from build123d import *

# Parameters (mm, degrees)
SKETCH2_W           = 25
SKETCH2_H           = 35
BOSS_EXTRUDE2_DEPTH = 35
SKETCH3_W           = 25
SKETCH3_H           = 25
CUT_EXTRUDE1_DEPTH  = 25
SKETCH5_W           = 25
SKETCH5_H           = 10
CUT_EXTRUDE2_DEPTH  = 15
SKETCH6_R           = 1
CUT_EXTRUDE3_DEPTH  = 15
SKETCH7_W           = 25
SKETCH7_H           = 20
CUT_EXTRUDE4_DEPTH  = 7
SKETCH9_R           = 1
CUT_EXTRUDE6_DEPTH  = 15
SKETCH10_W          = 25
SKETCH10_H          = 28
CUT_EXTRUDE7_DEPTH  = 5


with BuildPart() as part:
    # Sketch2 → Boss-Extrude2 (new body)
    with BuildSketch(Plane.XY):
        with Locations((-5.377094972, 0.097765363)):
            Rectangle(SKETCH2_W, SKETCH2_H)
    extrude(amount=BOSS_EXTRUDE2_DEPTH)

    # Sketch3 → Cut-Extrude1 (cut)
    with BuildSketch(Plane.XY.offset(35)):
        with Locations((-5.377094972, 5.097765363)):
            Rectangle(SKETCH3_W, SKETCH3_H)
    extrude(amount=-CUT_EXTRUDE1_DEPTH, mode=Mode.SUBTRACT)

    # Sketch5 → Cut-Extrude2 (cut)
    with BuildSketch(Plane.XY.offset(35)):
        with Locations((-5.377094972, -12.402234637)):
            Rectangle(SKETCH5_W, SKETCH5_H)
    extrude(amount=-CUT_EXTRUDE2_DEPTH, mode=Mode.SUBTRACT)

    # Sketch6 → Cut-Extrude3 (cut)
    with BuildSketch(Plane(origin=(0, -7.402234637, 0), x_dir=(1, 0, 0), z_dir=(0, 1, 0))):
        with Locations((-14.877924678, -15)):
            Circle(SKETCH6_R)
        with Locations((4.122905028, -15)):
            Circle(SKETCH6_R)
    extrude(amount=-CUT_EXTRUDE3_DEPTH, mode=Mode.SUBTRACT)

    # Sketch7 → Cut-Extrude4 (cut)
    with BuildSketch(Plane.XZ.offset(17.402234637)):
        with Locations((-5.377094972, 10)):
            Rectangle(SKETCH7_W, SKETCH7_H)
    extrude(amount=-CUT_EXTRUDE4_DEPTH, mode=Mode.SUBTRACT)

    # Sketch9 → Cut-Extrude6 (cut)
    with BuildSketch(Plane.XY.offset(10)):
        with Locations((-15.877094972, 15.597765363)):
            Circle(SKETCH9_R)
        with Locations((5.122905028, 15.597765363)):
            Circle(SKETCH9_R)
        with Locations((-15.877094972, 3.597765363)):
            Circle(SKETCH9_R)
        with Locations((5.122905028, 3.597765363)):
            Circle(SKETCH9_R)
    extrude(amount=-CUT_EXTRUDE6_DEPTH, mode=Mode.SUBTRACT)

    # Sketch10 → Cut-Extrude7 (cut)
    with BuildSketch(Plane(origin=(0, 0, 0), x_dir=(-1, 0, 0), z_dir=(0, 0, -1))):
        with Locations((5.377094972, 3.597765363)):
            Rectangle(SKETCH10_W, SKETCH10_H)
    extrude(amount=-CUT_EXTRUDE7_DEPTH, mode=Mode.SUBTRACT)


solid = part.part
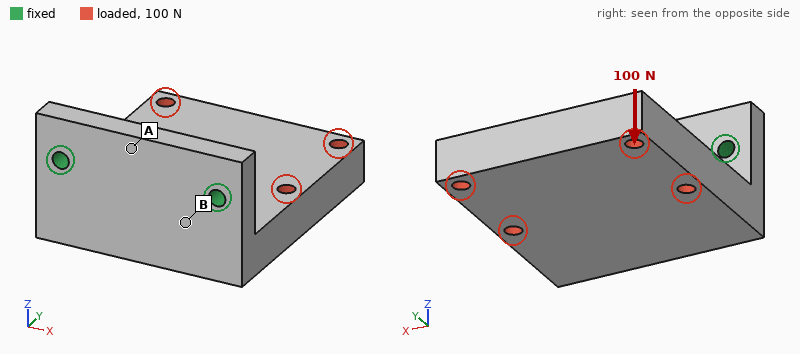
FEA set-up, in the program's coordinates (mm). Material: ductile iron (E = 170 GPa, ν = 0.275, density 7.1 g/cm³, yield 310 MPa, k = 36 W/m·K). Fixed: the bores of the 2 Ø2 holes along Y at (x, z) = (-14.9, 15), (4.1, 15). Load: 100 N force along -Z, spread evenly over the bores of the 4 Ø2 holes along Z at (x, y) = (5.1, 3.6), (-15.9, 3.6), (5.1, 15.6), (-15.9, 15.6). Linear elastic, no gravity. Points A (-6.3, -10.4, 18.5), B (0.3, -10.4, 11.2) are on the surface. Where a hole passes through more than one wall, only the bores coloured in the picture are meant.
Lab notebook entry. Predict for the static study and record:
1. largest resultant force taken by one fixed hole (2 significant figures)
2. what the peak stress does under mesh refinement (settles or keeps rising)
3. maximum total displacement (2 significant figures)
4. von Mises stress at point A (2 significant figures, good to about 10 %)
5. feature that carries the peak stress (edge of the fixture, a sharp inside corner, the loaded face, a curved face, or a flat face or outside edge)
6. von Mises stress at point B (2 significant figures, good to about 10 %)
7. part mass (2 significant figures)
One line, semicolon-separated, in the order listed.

52 N; keeps rising; 47 µm; 13 MPa; edge of the fixture; 40 MPa; 30 g
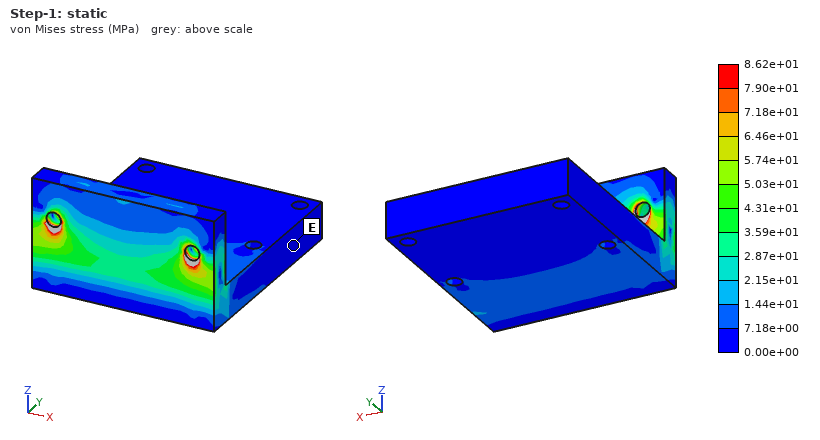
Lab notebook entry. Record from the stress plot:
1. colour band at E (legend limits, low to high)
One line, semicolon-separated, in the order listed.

0.00e+00 to 7.18e+00 MPa
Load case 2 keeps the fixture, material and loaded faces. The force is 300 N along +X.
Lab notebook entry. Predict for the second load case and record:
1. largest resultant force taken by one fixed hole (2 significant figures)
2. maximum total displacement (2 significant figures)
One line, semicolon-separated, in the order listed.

340 N; 16 µm
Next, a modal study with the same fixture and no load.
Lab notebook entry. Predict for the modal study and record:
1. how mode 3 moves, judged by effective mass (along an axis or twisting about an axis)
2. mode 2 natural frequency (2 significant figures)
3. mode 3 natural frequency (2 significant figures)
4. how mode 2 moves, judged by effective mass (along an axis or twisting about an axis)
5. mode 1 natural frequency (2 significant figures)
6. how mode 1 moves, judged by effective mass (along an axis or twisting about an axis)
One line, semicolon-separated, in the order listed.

along Y; 6300 Hz; 12 kHz; along X; 2200 Hz; along Z
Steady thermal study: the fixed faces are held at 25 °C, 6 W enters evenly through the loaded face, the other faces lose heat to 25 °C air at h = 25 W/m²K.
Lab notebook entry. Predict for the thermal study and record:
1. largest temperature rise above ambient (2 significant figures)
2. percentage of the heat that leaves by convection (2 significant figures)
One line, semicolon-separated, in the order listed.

40 K; 22 %
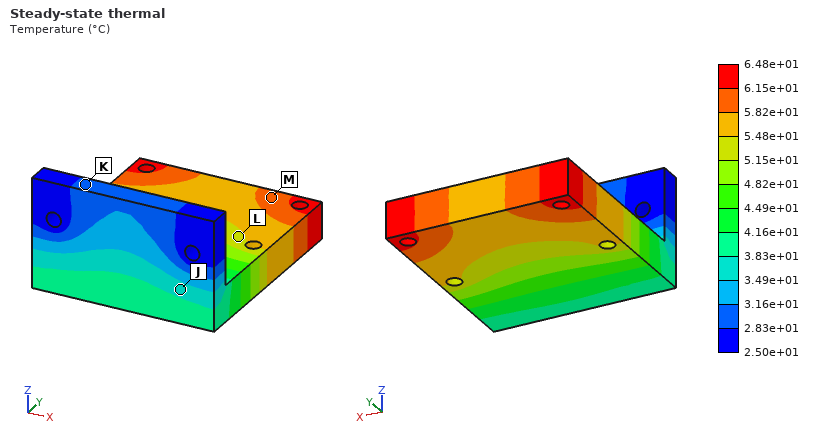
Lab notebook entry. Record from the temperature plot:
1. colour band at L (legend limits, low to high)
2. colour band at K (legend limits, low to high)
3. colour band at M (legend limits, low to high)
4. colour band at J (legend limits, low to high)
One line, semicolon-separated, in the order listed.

5.15e+01 to 5.48e+01 °C; 2.83e+01 to 3.16e+01 °C; 5.82e+01 to 6.15e+01 °C; 3.49e+01 to 3.83e+01 °C
